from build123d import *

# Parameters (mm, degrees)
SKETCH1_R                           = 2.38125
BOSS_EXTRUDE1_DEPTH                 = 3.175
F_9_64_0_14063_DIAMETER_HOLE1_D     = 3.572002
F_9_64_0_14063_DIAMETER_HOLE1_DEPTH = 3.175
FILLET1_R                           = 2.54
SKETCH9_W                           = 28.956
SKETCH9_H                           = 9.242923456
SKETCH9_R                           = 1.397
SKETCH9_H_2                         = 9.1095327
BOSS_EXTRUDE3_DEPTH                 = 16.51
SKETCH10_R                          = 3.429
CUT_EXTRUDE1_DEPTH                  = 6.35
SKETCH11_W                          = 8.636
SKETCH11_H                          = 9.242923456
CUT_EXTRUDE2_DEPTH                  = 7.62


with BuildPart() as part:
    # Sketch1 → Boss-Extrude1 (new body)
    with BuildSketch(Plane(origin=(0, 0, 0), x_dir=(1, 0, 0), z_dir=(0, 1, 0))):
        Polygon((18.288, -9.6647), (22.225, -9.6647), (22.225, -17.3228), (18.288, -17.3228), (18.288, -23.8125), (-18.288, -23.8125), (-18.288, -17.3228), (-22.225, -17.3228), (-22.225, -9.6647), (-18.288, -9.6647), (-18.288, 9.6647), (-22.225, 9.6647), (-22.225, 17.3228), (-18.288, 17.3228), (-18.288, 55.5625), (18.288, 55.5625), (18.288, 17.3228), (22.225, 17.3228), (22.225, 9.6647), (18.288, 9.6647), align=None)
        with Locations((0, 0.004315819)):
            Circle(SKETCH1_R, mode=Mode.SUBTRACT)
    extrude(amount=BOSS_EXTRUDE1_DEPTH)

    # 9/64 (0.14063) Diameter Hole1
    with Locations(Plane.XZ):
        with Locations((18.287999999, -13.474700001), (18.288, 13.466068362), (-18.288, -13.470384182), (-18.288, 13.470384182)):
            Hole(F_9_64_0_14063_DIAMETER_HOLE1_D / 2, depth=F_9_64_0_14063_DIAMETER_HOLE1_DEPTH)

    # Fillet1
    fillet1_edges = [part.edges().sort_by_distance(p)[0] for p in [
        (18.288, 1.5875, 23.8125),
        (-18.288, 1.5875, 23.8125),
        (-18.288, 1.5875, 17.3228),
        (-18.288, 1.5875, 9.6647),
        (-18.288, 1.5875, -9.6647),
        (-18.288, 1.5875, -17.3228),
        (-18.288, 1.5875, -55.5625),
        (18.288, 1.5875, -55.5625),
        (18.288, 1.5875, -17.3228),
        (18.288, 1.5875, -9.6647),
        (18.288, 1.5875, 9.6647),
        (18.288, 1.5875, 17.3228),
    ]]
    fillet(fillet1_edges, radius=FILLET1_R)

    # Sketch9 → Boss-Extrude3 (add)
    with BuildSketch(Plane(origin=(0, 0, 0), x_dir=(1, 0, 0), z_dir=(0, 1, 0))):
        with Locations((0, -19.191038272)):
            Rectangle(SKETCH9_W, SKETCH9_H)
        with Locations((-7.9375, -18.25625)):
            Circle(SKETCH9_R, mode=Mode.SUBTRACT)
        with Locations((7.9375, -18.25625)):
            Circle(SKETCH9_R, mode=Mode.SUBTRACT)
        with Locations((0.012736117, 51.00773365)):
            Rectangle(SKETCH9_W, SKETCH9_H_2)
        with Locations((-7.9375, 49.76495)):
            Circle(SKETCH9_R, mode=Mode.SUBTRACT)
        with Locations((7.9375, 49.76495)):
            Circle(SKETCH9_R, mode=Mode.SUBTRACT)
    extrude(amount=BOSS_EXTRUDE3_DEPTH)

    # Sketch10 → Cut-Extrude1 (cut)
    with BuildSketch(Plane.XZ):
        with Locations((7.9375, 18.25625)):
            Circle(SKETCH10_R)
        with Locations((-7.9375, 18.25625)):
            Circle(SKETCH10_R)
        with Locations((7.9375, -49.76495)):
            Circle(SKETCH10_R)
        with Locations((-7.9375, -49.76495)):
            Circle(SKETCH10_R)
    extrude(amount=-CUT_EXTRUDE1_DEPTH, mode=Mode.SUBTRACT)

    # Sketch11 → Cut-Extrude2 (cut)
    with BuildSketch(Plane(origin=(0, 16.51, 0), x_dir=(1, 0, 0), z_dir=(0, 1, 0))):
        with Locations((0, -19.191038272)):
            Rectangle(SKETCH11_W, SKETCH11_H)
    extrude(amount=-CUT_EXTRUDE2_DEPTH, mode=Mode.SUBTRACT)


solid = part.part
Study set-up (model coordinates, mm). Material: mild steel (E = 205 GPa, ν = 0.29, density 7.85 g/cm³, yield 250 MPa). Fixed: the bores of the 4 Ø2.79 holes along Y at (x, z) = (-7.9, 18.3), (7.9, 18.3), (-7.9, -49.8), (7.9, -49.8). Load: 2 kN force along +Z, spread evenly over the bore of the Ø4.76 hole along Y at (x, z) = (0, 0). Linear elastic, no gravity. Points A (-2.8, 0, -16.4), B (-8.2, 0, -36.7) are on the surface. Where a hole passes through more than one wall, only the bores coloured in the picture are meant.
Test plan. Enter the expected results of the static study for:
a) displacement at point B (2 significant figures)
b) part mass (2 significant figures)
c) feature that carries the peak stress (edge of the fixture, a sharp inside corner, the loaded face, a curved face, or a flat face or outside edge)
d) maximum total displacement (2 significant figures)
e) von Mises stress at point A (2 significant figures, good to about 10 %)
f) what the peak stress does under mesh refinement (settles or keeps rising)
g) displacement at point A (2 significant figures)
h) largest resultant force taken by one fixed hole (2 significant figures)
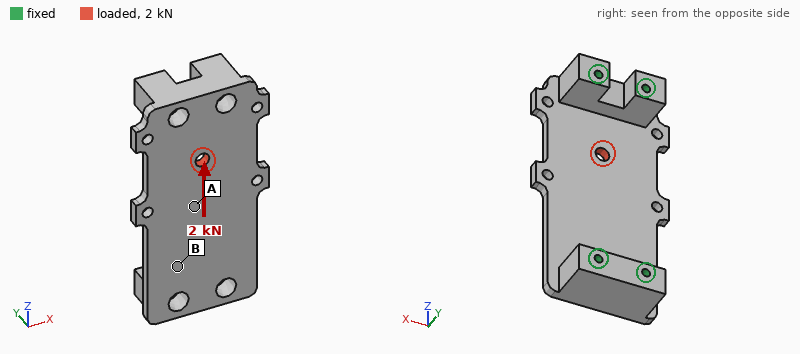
2.5 µm
120 g
edge of the fixture
5.6 µm
13 MPa
keeps rising
3.1 µm
590 N
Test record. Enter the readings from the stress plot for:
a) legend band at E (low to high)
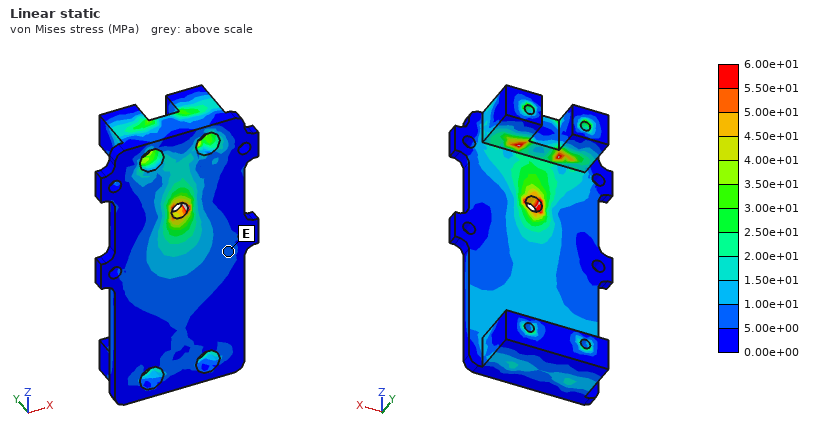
5.00e+00 to 1.00e+01 MPa
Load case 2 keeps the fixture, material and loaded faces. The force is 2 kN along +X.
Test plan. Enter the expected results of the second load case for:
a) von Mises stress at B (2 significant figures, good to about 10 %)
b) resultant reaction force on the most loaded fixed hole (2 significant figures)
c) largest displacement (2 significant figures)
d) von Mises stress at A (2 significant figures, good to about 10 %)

10 MPa
950 N
7.5 µm
9.8 MPa
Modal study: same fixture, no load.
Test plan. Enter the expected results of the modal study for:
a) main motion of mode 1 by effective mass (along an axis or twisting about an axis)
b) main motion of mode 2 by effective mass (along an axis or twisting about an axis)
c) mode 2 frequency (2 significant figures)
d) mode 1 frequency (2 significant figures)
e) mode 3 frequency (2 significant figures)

along Y
twisting about Z
5100 Hz
3600 Hz
9500 Hz
